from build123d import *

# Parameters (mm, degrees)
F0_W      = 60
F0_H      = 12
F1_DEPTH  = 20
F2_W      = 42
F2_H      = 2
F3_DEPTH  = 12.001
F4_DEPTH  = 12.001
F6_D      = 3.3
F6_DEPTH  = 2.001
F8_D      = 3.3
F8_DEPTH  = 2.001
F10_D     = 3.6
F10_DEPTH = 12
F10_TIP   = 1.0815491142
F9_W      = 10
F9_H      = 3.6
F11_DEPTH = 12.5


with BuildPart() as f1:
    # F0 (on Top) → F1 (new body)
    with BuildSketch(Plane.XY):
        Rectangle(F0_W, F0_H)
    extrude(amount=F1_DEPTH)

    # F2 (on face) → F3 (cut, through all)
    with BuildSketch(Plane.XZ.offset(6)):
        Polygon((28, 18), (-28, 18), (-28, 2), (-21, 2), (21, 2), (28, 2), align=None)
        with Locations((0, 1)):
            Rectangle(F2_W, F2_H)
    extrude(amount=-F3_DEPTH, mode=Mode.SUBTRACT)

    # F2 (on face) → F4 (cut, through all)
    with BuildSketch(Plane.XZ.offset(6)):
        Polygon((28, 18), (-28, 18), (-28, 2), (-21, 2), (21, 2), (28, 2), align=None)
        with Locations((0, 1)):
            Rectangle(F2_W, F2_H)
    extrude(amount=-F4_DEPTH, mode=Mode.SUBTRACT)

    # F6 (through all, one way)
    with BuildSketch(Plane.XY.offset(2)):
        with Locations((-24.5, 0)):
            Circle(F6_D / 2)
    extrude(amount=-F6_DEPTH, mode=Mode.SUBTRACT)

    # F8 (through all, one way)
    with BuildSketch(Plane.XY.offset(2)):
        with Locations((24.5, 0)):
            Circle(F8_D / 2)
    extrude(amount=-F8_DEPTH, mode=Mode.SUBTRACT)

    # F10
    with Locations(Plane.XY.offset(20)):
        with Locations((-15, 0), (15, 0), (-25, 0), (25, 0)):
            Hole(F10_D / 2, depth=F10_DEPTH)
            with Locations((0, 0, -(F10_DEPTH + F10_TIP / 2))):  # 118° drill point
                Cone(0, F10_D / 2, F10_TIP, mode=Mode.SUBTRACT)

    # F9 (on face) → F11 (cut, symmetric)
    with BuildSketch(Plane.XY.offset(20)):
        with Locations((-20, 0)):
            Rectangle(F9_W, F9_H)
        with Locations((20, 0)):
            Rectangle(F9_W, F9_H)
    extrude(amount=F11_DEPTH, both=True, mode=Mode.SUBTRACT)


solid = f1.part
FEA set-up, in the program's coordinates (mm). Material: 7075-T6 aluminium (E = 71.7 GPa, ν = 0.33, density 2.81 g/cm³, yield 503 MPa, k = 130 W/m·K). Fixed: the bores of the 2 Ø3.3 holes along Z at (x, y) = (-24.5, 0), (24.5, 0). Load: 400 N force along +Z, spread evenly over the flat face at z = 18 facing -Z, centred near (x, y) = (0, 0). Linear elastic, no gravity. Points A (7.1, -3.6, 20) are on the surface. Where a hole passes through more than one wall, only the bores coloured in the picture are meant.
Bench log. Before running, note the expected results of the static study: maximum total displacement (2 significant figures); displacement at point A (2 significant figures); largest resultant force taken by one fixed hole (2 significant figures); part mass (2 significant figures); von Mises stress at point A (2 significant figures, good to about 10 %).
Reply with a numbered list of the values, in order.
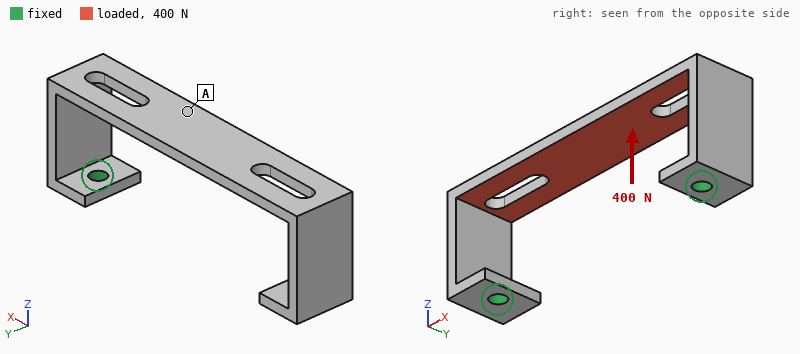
1. 0.67 mm
2. 0.60 mm
3. 230 N
4. 6.8 g
5. 160 MPa
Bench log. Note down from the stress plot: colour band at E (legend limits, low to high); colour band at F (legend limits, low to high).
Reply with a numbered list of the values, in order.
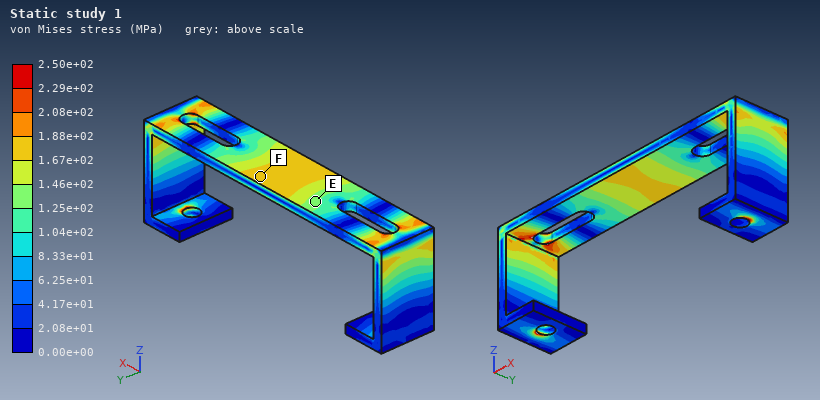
1. 1.25e+02 to 1.46e+02 MPa
2. 1.67e+02 to 1.88e+02 MPa
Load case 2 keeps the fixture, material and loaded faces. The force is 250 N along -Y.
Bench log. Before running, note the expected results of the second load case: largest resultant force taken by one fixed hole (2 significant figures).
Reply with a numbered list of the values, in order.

1. 130 N
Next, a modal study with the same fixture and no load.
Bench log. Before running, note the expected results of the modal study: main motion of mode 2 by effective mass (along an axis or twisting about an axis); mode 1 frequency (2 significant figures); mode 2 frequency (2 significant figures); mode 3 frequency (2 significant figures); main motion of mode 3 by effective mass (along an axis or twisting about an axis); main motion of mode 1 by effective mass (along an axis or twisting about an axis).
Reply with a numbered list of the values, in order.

1. along Z
2. 2100 Hz
3. 2400 Hz
4. 3000 Hz
5. along Y
6. along X
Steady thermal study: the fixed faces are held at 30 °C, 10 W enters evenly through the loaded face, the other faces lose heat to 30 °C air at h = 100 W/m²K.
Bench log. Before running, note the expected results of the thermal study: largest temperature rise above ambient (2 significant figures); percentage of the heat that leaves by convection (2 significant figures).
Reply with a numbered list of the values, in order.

1. 42 K
2. 45 %
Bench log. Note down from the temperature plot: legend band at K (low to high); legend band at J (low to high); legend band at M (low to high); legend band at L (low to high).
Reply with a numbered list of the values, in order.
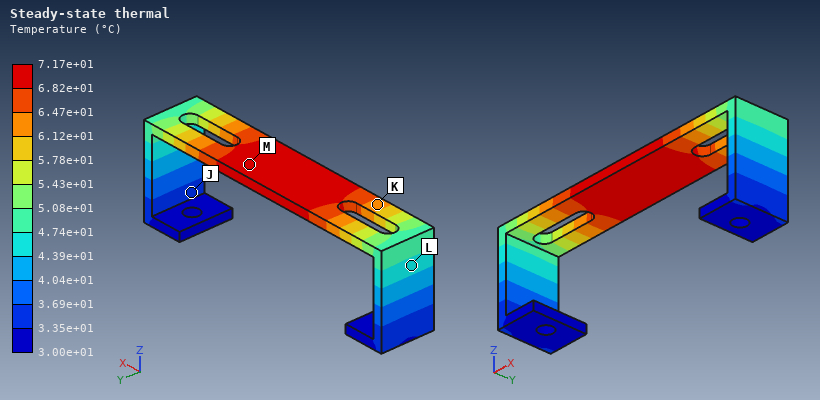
1. 6.12e+01 to 6.47e+01 °C
2. 3.35e+01 to 3.69e+01 °C
3. 6.82e+01 to 7.17e+01 °C
4. 4.39e+01 to 4.74e+01 °C
